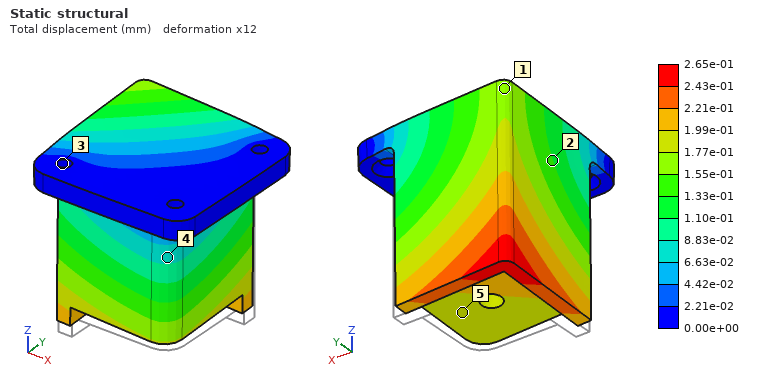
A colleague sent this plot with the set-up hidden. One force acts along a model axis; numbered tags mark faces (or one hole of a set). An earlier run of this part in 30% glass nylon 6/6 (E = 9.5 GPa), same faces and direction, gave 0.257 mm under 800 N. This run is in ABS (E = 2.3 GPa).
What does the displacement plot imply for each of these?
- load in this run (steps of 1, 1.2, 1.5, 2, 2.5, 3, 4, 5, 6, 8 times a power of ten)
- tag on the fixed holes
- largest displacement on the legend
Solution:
200 N
3
2.65e-01 mm
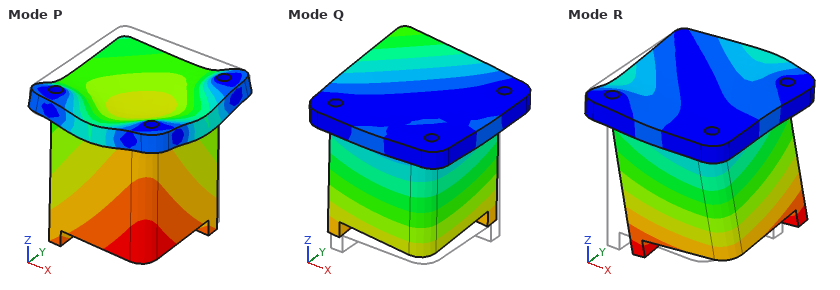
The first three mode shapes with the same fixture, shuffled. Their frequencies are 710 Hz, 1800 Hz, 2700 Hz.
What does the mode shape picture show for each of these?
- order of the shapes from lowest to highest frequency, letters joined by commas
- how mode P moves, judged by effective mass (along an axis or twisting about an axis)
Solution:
Q, R, P
along Z
